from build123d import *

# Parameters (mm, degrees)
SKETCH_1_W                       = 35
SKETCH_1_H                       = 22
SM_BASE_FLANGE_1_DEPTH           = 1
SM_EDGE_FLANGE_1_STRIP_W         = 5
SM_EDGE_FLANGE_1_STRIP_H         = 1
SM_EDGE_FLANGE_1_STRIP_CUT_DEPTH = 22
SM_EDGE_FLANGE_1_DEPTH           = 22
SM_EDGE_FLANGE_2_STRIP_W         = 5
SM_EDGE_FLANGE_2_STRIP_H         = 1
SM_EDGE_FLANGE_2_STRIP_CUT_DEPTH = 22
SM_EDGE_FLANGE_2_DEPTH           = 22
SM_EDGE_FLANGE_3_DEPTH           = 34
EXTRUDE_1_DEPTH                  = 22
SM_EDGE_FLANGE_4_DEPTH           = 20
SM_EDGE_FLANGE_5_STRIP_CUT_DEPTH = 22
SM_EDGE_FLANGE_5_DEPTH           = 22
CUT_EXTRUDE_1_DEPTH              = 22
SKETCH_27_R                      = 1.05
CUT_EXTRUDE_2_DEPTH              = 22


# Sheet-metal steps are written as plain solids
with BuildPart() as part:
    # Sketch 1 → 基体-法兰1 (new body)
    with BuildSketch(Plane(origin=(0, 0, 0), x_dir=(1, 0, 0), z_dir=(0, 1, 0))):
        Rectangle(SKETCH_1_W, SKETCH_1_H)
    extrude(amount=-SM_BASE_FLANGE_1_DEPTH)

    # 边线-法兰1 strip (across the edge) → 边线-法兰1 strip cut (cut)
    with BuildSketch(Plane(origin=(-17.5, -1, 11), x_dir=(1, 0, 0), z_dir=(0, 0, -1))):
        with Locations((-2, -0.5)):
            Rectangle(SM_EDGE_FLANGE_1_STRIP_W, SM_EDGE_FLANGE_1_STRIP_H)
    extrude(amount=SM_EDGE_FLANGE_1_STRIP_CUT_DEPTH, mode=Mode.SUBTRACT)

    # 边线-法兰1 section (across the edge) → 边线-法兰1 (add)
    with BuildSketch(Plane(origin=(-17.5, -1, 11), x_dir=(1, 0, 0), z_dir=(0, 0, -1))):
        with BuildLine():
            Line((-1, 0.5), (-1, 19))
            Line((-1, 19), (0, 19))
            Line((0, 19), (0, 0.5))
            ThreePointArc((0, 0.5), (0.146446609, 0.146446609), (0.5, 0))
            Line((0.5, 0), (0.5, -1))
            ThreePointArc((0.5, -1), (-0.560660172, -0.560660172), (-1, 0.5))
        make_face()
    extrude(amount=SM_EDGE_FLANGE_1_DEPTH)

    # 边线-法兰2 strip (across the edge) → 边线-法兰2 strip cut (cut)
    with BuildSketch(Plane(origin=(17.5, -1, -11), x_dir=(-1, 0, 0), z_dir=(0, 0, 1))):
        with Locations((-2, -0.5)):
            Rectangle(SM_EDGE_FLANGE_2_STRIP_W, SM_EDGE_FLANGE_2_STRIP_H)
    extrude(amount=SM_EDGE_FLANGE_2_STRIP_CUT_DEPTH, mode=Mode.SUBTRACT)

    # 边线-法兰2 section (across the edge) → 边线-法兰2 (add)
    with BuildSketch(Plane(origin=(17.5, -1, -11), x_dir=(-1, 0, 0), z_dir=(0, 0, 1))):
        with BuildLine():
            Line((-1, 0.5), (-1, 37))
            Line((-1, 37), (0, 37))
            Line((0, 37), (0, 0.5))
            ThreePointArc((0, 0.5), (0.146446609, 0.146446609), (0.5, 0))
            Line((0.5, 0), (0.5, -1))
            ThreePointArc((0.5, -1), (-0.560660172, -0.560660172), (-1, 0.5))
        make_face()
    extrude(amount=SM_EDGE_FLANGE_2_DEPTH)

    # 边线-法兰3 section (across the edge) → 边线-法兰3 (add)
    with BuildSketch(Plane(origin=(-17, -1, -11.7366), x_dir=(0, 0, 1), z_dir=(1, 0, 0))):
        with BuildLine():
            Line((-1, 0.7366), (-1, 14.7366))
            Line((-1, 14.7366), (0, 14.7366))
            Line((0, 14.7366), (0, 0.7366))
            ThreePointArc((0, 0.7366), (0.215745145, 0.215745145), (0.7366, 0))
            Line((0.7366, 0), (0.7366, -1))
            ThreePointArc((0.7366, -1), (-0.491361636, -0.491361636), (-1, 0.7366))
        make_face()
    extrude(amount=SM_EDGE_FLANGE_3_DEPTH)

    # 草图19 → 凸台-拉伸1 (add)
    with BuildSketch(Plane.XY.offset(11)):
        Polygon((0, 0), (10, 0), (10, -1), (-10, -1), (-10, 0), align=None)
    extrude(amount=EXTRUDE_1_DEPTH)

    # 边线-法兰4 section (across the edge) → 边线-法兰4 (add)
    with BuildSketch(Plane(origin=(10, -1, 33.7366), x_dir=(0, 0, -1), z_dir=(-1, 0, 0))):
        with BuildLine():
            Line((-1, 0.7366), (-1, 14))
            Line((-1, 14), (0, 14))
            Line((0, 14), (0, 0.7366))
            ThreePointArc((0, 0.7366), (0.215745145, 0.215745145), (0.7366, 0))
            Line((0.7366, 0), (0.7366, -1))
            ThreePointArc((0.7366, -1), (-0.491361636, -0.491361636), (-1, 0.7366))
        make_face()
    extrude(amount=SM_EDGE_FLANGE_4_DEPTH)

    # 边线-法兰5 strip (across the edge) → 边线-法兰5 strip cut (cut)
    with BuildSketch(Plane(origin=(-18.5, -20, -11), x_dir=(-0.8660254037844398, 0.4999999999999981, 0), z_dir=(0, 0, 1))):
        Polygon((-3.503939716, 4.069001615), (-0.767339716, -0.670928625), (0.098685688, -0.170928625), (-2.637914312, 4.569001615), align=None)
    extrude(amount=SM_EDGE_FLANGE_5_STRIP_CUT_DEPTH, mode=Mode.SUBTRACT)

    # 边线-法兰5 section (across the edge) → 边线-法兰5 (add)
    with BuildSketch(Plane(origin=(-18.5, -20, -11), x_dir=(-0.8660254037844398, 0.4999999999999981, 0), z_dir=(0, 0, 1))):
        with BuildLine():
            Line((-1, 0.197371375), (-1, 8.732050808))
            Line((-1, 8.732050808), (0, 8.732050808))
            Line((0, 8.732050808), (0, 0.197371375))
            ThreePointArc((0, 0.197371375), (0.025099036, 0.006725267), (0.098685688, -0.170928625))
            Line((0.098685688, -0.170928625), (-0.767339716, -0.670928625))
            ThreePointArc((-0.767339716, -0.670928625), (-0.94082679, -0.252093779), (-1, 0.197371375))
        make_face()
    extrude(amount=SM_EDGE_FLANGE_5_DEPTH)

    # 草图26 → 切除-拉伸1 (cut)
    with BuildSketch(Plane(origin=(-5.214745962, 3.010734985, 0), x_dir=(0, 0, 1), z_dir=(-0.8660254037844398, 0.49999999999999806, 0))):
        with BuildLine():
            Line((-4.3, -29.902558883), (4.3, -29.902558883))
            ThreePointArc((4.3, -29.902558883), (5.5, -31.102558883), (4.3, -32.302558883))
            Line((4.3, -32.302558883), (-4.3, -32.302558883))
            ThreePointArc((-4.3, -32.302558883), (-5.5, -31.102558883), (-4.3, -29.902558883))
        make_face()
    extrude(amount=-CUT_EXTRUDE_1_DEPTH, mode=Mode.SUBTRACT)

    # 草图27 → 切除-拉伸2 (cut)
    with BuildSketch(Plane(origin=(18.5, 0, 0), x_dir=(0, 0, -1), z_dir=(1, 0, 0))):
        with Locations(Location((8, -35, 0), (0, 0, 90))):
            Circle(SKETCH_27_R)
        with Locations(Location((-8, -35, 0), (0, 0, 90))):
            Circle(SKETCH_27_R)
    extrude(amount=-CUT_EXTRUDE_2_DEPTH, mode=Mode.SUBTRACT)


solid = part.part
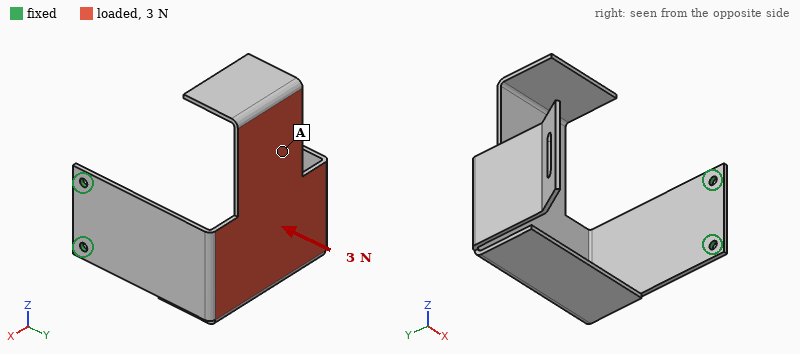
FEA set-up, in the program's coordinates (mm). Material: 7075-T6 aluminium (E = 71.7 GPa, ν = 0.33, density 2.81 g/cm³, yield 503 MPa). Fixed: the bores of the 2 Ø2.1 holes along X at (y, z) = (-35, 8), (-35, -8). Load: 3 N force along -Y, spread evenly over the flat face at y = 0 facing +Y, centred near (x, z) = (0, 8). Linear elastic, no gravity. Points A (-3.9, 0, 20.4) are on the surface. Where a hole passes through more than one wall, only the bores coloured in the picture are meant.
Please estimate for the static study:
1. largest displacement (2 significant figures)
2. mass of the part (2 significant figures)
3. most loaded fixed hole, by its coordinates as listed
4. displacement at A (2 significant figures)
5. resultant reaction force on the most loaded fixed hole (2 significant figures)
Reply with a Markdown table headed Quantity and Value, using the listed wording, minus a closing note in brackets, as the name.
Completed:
| Quantity | Value |
|---|---|
| largest displacement | 0.67 mm |
| mass of the part | 9.8 g |
| most loaded fixed hole, by its coordinates as listed | (-35, 8) |
| displacement at A | 0.44 mm |
| resultant reaction force on the most loaded fixed hole | 3.0 N |
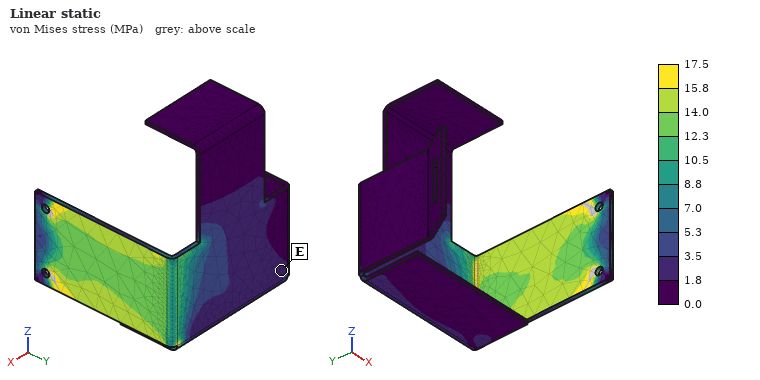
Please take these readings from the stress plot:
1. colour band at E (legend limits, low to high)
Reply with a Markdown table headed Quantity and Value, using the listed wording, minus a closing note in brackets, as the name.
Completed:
| Quantity | Value |
|---|---|
| colour band at E | 1.8 to 3.5 MPa |
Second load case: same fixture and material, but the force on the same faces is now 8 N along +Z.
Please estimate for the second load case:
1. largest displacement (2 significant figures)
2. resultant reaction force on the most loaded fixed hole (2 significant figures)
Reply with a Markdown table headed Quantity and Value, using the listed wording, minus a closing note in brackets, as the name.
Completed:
| Quantity | Value |
|---|---|
| largest displacement | 0.87 mm |
| resultant reaction force on the most loaded fixed hole | 19 N |
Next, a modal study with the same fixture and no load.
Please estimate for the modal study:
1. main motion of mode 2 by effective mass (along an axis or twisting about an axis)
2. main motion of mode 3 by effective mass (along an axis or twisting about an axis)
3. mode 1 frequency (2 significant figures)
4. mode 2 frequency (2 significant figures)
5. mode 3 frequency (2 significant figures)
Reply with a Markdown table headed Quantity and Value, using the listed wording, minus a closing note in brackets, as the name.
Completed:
| Quantity | Value |
|---|---|
| main motion of mode 2 by effective mass | along Z |
| main motion of mode 3 by effective mass | along X |
| mode 1 frequency | 120 Hz |
| mode 2 frequency | 170 Hz |
| mode 3 frequency | 320 Hz |
